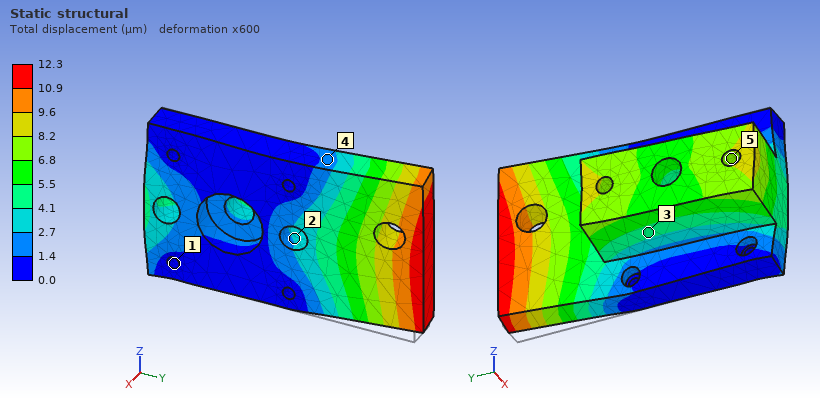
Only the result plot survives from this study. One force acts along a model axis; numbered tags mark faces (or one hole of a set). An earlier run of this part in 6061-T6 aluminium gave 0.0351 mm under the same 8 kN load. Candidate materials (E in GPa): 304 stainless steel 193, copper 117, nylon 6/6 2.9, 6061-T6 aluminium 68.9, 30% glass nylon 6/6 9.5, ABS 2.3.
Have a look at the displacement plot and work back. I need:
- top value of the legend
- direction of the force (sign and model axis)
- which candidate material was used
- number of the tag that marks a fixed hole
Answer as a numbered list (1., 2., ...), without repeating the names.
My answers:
1. 12.3 µm
2. -Y
3. 304 stainless steel
4. 1
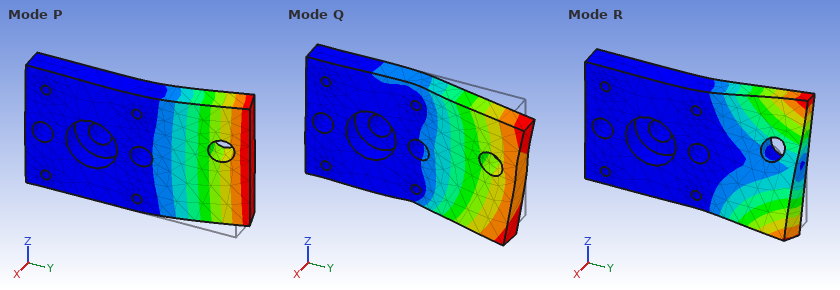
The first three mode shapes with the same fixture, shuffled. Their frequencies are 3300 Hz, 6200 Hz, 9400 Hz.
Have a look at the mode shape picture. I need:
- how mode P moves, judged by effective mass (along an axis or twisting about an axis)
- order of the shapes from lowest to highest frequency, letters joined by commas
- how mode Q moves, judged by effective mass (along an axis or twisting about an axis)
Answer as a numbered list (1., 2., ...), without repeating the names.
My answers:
1. along X
2. P, R, Q
3. along Z
